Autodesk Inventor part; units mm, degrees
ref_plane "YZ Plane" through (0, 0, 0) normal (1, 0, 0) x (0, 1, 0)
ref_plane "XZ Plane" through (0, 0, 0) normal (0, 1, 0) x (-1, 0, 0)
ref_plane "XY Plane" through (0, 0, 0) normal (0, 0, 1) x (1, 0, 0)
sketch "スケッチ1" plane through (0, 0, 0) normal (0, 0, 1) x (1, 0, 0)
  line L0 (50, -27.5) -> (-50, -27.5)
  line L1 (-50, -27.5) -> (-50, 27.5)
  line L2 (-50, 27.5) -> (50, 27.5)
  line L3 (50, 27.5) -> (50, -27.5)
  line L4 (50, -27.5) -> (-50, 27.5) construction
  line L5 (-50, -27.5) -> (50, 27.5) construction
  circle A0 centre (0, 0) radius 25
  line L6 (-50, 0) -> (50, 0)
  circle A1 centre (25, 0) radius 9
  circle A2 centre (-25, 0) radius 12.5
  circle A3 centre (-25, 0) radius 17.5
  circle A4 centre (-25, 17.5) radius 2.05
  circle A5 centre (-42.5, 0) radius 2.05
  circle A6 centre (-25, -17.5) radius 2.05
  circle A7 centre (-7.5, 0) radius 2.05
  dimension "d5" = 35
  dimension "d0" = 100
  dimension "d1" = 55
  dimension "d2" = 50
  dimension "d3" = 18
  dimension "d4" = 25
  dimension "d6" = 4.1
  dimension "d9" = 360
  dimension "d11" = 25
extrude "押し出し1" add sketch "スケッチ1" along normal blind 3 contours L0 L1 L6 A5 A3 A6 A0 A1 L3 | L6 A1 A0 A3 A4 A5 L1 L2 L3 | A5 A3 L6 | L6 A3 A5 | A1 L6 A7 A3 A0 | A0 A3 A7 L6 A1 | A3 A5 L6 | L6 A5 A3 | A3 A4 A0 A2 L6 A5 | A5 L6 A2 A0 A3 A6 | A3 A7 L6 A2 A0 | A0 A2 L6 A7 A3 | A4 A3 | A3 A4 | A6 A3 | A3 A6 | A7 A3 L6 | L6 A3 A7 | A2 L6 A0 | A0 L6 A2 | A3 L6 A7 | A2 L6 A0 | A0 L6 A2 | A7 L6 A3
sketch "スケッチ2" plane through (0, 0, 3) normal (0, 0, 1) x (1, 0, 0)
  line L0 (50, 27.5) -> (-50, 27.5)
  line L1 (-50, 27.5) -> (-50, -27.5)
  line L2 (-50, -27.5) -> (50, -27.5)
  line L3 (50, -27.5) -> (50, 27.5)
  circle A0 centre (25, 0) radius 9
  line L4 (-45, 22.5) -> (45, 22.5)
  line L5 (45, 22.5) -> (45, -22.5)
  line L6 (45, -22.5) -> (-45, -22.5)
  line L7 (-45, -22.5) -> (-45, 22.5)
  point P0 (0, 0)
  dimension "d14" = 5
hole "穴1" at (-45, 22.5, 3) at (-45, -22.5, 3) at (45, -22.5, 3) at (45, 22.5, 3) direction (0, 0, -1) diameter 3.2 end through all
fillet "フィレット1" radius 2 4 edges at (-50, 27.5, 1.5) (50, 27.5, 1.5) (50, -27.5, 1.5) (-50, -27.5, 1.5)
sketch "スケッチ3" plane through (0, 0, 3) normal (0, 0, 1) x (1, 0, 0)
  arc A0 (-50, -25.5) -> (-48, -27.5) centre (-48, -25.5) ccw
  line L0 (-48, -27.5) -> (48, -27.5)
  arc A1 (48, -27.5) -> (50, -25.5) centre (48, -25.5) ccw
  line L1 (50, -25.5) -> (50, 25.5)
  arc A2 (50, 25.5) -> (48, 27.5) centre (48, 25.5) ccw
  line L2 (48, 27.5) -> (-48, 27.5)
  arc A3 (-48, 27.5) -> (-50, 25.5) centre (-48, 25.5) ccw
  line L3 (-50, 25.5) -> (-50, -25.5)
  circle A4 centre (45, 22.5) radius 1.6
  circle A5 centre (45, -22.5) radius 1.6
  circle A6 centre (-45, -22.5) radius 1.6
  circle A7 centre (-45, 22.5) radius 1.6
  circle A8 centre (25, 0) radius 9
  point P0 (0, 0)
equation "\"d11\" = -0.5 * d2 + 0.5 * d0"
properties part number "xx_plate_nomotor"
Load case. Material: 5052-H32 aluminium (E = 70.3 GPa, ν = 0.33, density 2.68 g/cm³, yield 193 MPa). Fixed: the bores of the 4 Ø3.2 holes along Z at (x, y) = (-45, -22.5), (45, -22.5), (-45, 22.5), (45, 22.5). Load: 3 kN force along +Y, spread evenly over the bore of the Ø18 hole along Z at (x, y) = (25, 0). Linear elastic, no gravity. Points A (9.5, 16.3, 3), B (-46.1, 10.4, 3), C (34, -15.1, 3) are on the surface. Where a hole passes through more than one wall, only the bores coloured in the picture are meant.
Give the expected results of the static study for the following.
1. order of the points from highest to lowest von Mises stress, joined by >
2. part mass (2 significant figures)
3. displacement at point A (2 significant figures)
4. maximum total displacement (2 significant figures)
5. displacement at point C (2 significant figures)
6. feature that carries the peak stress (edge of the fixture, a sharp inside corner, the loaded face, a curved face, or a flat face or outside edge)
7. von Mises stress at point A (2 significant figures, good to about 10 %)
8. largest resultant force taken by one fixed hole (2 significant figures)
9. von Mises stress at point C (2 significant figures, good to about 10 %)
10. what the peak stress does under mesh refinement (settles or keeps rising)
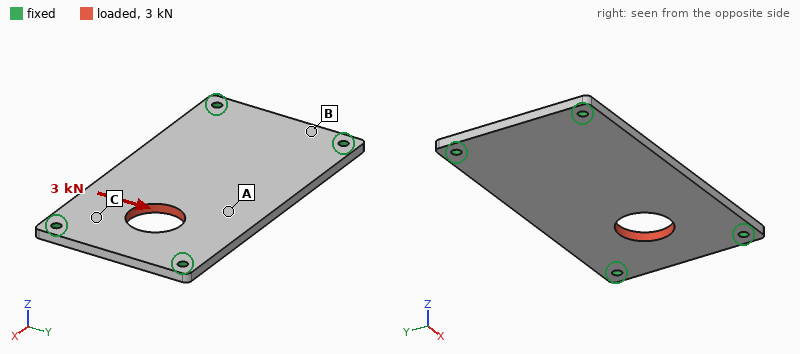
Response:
C > A > B
42 g
18 µm
22 µm
10 µm
edge of the fixture
11 MPa
1.2 kN
25 MPa
keeps rising
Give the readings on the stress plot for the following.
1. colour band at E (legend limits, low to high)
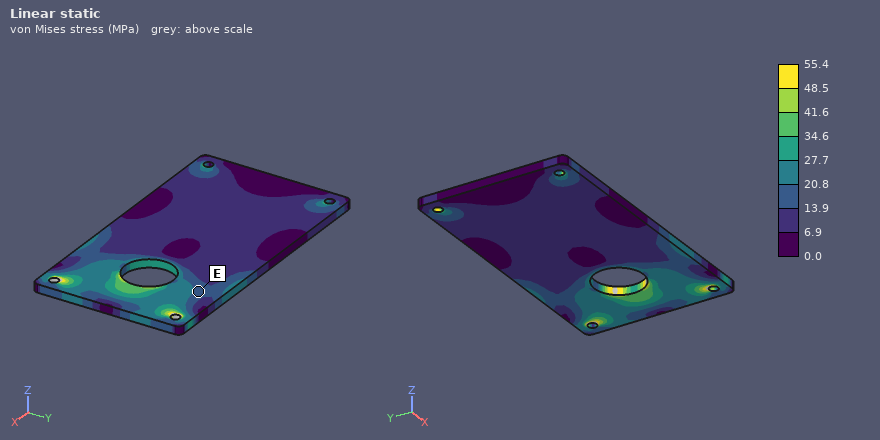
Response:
13.9 to 20.8 MPa
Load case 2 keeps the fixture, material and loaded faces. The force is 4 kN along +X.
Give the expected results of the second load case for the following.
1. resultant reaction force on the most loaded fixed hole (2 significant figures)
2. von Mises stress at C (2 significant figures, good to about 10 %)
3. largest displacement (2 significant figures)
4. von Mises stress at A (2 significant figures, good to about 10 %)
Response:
1.4 kN
23 MPa
19 µm
13 MPa
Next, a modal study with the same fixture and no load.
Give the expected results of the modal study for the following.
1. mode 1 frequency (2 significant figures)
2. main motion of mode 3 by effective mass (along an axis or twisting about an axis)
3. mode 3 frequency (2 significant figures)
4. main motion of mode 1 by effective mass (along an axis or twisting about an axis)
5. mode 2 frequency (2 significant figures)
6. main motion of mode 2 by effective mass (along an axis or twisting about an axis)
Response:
1700 Hz
twisting about Y
4700 Hz
along Z
2800 Hz
twisting about X
